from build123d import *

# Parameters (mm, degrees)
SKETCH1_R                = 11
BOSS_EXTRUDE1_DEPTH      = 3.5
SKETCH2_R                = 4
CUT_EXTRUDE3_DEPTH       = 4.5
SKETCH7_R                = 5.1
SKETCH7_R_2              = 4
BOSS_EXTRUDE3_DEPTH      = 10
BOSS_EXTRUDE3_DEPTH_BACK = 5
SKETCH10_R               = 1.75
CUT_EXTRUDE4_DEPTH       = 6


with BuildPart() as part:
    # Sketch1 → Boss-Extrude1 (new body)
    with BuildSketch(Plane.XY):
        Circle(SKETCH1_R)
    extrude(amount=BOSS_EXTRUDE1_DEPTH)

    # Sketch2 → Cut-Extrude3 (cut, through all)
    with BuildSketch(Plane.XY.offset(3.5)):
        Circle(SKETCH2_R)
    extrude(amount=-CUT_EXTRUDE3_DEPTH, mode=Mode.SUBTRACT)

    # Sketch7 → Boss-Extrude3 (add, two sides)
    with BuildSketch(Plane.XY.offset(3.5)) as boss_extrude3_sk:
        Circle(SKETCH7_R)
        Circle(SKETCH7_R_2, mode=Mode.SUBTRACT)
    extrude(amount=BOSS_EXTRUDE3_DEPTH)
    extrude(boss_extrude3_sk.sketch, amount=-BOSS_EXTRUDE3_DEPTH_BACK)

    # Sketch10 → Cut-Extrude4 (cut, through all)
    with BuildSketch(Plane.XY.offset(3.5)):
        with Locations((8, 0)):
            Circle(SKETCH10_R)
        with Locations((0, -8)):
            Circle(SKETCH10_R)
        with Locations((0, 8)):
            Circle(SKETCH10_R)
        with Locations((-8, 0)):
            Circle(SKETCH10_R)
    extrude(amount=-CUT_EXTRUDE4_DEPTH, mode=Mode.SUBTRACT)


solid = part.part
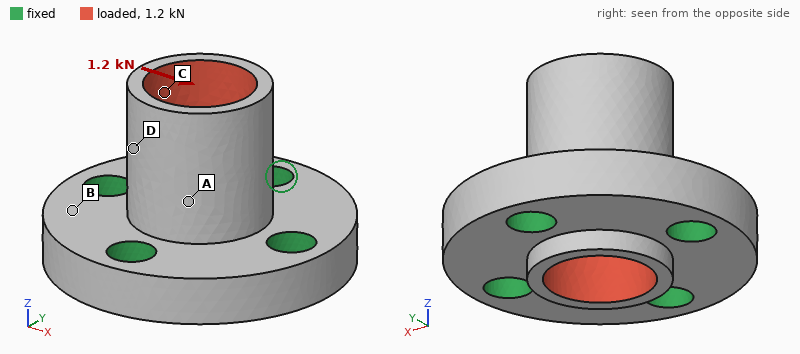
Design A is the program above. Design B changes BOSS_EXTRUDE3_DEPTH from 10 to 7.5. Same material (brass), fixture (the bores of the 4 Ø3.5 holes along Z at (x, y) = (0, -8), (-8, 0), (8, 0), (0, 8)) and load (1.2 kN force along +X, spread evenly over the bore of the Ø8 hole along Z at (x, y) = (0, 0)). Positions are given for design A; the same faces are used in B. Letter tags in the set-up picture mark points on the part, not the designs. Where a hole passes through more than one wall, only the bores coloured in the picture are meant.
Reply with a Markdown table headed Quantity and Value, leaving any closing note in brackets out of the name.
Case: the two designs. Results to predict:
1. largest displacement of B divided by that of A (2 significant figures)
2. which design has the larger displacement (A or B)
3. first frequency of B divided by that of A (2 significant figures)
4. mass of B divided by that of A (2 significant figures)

| Quantity | Value |
|---|---|
| largest displacement of B divided by that of A | 0.61 |
| which design has the larger displacement | A |
| first frequency of B divided by that of A | 1.3 |
| mass of B divided by that of A | 0.94 |
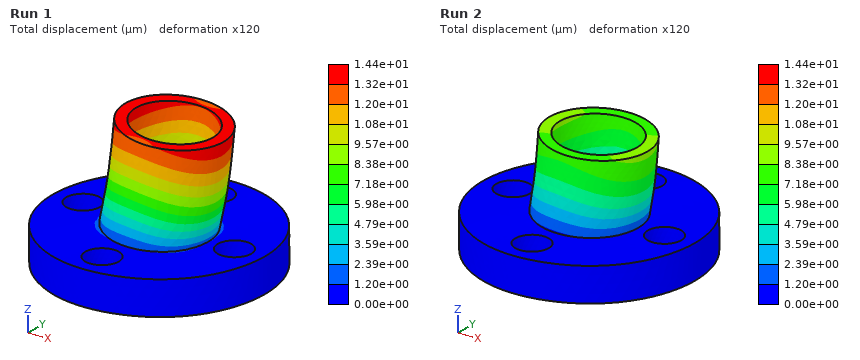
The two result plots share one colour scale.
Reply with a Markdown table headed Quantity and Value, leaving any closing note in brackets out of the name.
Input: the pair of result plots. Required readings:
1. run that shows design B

| Quantity | Value |
|---|---|
| run that shows design B | Run 2 |
